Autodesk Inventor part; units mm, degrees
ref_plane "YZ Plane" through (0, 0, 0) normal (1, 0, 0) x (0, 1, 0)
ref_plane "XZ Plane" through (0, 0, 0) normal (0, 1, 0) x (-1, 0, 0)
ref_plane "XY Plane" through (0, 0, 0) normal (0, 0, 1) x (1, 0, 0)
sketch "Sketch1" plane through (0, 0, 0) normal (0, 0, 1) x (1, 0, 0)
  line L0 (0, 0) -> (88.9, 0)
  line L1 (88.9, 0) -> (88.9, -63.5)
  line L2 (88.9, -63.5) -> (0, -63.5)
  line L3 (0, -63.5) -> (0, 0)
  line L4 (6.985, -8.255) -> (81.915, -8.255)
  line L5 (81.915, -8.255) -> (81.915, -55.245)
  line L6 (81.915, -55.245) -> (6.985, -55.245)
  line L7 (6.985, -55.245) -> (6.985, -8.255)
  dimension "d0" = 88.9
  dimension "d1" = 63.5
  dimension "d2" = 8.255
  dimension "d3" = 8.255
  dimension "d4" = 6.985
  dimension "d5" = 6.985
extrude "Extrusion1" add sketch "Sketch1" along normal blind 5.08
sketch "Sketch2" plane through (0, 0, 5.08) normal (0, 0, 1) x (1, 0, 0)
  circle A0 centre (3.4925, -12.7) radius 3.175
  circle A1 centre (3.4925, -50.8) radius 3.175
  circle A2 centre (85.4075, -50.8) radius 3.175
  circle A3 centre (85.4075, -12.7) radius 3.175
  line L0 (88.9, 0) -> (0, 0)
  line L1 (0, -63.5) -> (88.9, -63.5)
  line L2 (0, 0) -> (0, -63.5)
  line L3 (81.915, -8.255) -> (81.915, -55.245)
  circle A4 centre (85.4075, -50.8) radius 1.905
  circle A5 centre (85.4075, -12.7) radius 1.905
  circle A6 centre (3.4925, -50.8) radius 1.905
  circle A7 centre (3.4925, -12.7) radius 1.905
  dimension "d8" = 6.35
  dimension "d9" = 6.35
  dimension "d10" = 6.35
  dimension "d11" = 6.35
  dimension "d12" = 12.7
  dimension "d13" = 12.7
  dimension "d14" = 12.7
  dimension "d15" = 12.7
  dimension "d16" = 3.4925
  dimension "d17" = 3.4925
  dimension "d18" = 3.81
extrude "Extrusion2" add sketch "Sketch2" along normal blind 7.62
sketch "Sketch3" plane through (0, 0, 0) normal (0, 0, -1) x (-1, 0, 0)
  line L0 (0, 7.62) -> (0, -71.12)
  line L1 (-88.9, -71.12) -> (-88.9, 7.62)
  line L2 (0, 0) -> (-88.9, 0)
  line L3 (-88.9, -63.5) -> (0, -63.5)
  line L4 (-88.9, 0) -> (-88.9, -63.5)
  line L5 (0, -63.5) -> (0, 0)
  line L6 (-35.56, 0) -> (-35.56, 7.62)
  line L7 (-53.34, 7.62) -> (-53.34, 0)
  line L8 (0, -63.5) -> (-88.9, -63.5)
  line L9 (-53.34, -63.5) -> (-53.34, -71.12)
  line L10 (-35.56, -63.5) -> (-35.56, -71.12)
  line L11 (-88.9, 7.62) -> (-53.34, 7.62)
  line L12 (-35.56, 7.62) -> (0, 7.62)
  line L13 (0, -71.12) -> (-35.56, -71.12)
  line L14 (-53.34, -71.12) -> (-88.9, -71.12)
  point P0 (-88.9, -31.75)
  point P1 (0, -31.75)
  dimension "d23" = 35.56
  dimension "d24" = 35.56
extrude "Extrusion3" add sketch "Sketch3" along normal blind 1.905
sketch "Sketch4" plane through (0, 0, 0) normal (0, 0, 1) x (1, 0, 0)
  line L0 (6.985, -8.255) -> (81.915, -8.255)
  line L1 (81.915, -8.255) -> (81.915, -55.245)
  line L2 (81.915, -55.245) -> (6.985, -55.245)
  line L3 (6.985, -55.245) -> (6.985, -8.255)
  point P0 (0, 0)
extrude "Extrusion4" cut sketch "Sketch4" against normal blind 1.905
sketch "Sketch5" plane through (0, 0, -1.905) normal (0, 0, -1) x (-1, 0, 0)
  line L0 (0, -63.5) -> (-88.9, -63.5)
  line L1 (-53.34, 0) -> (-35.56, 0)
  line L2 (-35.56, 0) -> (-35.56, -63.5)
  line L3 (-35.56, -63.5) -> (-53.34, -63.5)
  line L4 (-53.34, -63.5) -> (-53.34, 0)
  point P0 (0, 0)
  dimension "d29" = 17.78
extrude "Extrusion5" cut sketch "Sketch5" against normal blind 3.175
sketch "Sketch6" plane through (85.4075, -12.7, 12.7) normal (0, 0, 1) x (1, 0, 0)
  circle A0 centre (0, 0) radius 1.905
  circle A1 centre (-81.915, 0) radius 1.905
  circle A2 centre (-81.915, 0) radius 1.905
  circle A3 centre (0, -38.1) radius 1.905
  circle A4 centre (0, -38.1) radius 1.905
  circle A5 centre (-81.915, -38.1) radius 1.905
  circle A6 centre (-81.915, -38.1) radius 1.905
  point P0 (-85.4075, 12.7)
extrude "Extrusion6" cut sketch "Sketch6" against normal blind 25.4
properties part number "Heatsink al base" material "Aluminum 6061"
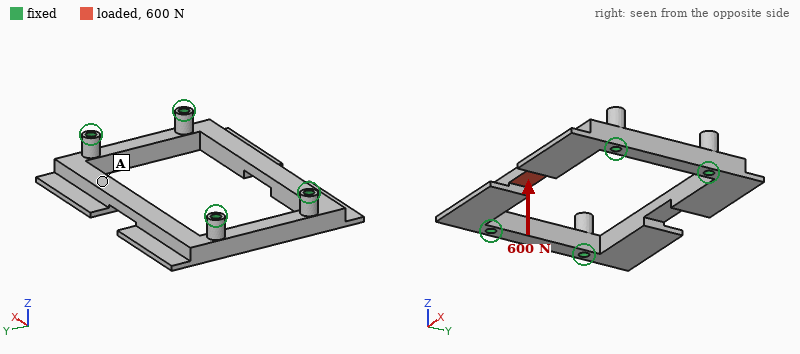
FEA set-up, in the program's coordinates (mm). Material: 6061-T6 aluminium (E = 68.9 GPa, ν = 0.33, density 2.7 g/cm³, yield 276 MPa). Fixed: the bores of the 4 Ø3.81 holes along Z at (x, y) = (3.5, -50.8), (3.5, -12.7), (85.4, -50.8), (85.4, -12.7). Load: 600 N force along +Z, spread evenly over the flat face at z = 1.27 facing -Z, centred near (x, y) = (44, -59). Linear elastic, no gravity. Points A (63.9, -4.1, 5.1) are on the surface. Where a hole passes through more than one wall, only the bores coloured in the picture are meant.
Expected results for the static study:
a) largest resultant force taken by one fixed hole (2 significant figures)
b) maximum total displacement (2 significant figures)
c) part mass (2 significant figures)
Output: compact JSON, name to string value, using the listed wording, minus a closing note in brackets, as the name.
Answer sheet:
{"largest resultant force taken by one fixed hole": "550 N", "maximum total displacement": "0.29 mm", "part mass": "44 g"}
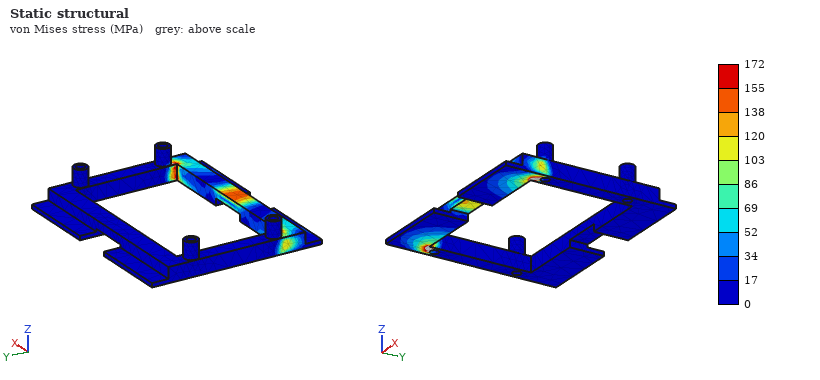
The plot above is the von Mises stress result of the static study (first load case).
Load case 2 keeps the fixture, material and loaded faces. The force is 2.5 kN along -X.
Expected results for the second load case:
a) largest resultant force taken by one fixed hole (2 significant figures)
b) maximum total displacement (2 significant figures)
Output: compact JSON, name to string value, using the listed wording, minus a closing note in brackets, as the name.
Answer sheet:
{"largest resultant force taken by one fixed hole": "1.3 kN", "maximum total displacement": "39 µm"}
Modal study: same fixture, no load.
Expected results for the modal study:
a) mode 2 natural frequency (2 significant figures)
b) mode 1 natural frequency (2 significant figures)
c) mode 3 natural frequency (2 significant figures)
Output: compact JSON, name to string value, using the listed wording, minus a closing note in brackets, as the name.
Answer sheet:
{"mode 2 natural frequency": "3400 Hz", "mode 1 natural frequency": "3400 Hz", "mode 3 natural frequency": "5100 Hz"}
